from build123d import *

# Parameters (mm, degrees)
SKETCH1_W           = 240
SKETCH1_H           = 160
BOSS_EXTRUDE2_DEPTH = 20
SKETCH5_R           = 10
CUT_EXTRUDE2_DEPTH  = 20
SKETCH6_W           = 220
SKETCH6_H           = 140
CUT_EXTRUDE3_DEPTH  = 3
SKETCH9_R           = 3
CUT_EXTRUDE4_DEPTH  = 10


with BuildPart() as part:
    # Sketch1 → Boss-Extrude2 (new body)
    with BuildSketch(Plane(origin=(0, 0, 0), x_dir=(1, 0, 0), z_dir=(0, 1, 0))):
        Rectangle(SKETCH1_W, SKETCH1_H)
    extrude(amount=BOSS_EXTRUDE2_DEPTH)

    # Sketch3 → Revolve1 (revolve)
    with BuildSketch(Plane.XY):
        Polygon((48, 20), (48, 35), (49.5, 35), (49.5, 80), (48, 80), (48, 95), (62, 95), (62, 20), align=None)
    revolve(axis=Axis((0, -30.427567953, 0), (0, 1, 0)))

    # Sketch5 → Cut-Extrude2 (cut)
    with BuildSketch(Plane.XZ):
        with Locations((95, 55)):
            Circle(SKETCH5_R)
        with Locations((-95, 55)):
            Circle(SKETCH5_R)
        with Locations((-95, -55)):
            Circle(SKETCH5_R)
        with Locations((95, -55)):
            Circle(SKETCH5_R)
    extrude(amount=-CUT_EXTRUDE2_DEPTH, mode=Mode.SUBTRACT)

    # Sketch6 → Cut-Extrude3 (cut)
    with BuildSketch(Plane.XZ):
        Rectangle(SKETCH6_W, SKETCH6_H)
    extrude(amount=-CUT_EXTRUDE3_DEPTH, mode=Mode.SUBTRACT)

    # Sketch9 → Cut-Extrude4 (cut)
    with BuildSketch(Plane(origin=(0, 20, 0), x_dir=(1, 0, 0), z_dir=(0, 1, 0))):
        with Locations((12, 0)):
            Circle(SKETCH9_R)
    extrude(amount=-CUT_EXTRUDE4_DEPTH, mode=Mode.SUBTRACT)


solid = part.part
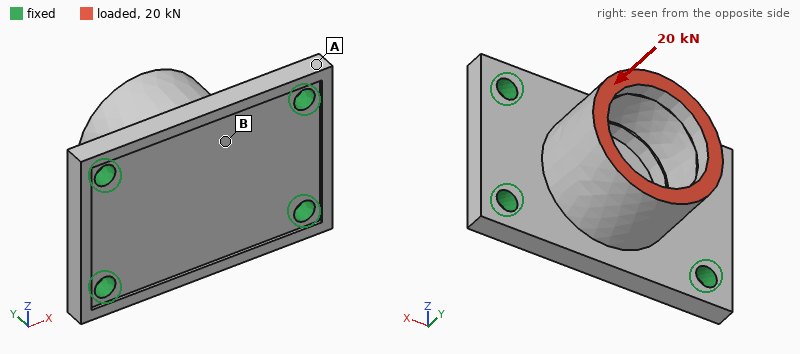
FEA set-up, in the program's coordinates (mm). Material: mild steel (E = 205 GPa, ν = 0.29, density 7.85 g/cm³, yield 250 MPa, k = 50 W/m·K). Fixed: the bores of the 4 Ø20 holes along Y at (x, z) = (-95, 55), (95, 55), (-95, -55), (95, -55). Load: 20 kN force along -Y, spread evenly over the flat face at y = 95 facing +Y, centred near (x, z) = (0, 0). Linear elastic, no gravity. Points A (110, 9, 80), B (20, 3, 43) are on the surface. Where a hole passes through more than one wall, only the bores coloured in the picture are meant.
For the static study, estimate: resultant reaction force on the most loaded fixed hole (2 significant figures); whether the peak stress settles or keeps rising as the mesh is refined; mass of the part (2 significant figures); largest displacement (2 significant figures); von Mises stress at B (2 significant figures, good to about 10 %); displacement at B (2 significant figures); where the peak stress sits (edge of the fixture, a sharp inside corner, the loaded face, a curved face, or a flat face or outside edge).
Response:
5.2 kN
keeps rising
7.8 kg
21 µm
9.0 MPa
18 µm
edge of the fixture
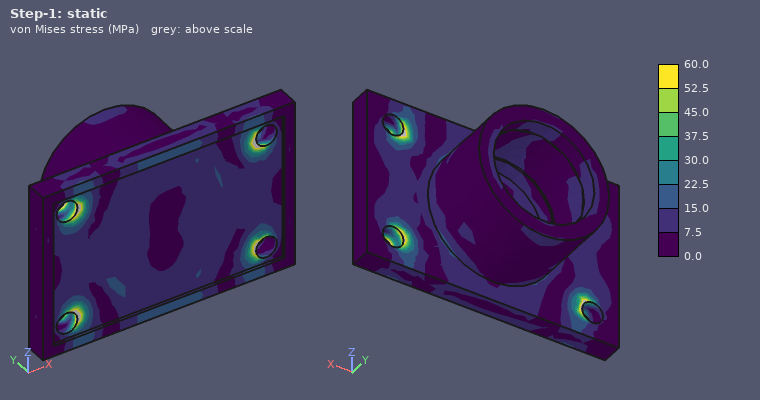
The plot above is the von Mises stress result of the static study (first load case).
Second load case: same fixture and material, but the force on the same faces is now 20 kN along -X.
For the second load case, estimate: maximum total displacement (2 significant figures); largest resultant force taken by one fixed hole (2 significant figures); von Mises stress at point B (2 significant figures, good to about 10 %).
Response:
39 µm
7.6 kN
8.6 MPa
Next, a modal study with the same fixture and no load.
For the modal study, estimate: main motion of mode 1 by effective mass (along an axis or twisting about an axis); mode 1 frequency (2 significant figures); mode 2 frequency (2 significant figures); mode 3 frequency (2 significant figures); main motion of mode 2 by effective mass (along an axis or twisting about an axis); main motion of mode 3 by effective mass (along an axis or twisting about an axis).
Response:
along Z
2100 Hz
2300 Hz
3300 Hz
along Y
along X
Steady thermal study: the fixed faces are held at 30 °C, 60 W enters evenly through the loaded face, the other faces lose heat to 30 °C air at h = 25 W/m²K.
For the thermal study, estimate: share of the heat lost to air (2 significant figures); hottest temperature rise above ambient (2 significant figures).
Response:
47 %
23 K
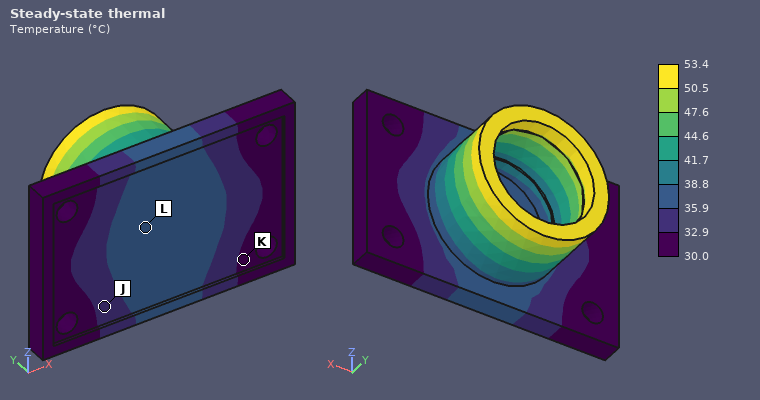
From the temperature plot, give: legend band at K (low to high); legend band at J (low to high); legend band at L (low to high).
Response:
30.0 to 32.9 °C
32.9 to 35.9 °C
35.9 to 38.8 °C
